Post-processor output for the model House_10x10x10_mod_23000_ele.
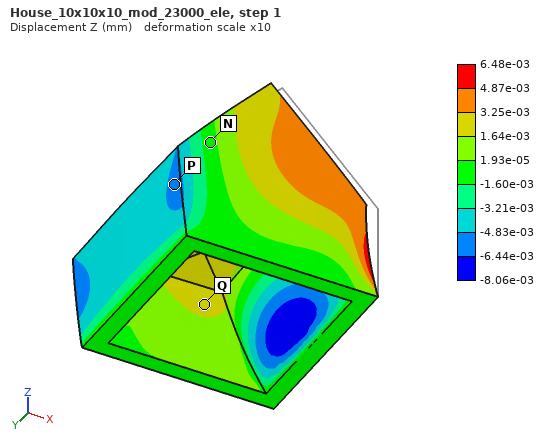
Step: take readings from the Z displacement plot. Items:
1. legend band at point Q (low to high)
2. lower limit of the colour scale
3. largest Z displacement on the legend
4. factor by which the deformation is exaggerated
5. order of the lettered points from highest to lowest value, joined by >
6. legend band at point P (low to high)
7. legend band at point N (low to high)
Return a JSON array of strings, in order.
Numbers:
["1.64e-03 to 3.25e-03 mm", "-8.06e-03 mm", "6.48e-03 mm", "10", "Q > N > P", "-6.44e-03 to -4.83e-03 mm", "-1.60e-03 to 1.93e-05 mm"]
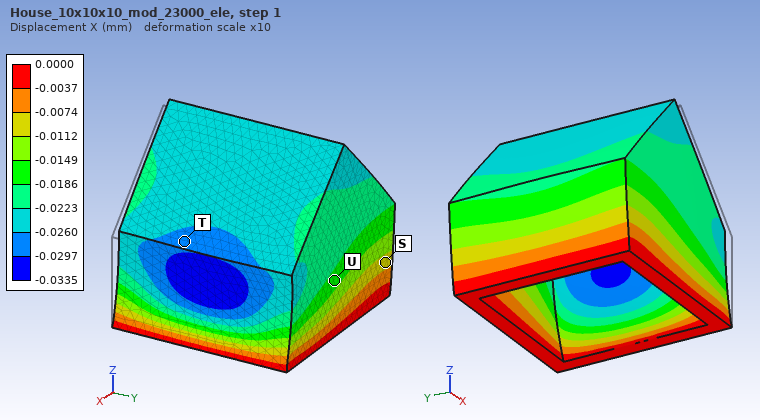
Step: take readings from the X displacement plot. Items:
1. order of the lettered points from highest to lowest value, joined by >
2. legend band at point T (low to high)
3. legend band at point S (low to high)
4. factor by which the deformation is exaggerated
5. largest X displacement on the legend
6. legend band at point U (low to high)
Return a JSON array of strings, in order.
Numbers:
["S > U > T", "-0.0297 to -0.0260 mm", "-0.0112 to -0.0074 mm", "10", "0.0000 mm", "-0.0186 to -0.0149 mm"]
